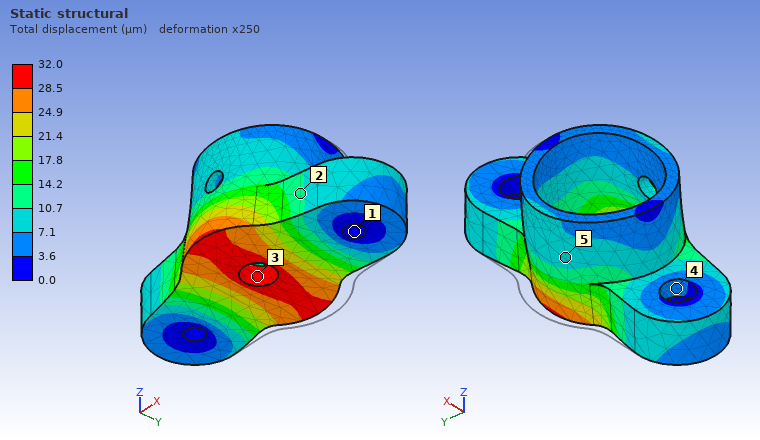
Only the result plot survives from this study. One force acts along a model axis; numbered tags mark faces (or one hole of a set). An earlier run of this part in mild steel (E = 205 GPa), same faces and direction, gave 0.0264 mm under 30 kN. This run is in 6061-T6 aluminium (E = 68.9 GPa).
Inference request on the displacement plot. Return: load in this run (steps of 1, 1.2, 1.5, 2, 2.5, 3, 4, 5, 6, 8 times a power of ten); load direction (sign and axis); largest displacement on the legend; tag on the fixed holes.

12 kN
-Y
32.0 µm
1
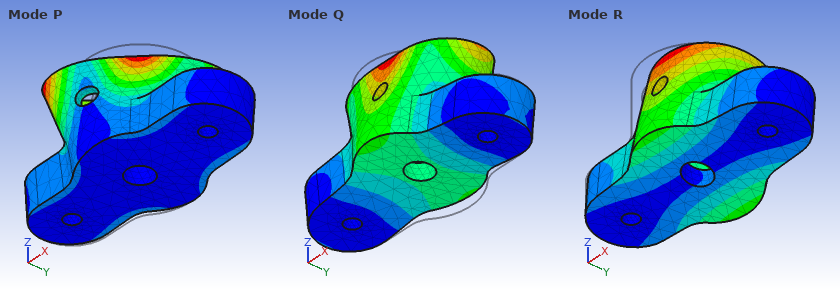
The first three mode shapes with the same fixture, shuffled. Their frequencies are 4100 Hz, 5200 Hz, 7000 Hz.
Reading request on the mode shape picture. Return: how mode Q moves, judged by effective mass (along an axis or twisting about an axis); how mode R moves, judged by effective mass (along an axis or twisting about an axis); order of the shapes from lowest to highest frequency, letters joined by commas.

along Z
along Y
R, Q, P
